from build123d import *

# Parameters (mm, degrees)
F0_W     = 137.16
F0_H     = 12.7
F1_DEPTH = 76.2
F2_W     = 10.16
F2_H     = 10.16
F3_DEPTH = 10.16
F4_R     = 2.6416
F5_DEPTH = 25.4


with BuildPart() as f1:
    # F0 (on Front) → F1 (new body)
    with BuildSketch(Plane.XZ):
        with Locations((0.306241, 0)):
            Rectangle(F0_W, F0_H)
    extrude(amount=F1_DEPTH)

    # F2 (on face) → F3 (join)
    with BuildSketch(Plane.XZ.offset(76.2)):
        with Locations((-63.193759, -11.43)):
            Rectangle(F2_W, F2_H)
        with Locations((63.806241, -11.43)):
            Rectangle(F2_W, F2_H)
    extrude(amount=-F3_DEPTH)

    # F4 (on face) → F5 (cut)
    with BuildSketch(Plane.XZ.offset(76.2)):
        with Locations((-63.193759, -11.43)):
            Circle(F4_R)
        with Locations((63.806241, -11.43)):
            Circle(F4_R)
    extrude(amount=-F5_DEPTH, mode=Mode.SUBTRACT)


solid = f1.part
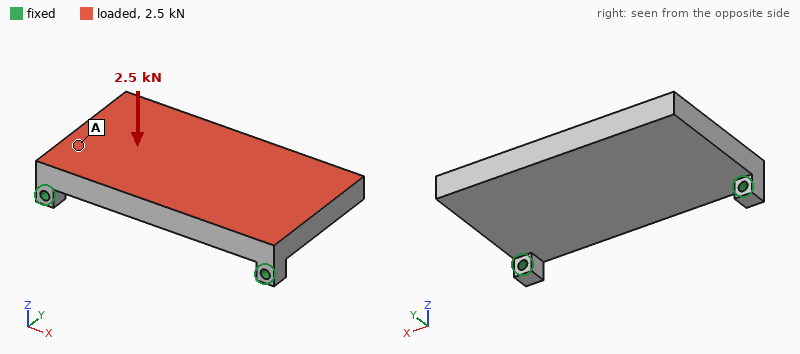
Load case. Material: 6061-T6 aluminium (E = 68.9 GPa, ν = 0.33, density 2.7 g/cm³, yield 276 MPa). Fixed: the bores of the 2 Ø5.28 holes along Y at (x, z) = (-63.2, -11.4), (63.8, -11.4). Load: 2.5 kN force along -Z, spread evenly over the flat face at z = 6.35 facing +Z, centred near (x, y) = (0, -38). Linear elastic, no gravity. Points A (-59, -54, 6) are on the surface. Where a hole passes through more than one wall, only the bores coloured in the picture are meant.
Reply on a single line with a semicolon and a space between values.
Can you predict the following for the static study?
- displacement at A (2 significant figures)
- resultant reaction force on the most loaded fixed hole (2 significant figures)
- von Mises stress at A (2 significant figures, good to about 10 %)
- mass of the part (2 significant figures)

0.13 mm; 1.6 kN; 29 MPa; 360 g
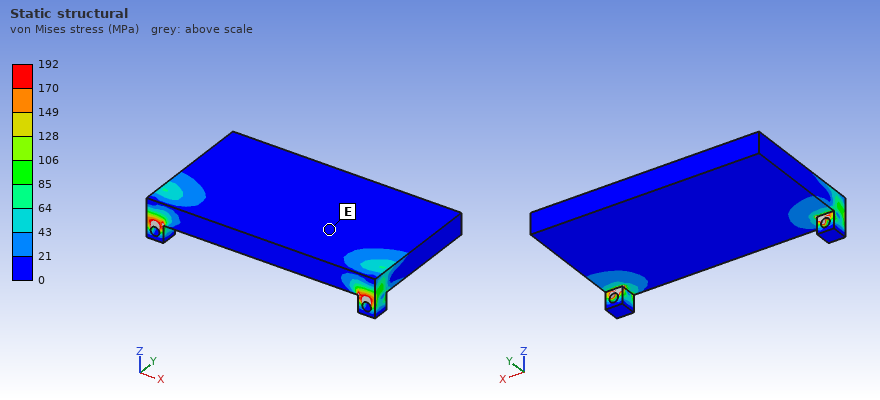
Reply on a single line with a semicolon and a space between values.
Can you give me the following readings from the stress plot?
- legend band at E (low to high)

0 to 21 MPa
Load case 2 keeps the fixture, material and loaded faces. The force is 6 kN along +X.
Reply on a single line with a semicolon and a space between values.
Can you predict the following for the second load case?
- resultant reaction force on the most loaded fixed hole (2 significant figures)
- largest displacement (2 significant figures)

3.4 kN; 32 µm
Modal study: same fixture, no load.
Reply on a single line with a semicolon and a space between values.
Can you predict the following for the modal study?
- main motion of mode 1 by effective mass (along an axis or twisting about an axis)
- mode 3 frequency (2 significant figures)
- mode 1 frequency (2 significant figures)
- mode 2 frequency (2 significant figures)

along Z; 3200 Hz; 690 Hz; 2300 Hz
